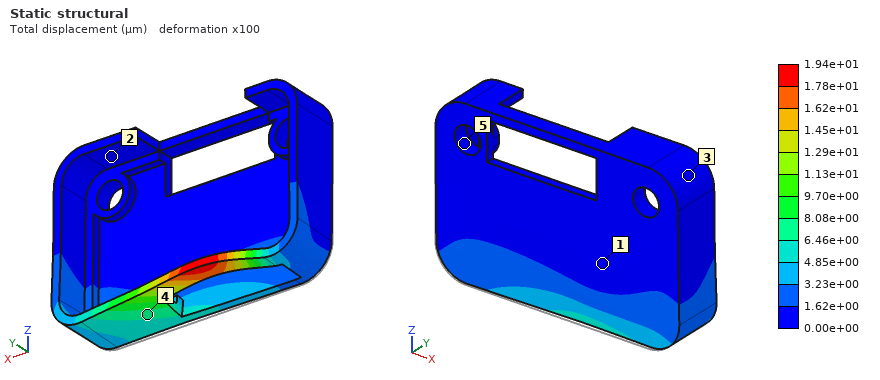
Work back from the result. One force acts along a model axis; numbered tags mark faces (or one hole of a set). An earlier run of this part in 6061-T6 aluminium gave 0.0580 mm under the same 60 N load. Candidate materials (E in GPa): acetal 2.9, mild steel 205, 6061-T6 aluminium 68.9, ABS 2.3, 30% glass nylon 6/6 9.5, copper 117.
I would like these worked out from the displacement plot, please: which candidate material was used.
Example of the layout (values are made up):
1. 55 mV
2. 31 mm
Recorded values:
1. mild steel
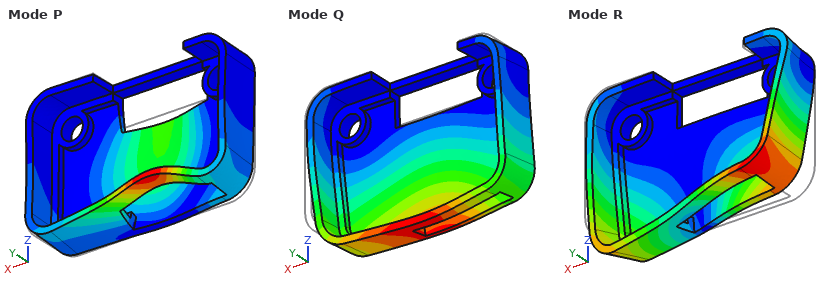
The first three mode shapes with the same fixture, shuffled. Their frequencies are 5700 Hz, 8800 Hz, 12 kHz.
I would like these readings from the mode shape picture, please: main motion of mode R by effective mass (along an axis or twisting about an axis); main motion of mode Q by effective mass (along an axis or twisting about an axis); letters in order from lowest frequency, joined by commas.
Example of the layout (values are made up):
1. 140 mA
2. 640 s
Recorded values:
1. twisting about Z
2. along Y
3. Q, R, P
